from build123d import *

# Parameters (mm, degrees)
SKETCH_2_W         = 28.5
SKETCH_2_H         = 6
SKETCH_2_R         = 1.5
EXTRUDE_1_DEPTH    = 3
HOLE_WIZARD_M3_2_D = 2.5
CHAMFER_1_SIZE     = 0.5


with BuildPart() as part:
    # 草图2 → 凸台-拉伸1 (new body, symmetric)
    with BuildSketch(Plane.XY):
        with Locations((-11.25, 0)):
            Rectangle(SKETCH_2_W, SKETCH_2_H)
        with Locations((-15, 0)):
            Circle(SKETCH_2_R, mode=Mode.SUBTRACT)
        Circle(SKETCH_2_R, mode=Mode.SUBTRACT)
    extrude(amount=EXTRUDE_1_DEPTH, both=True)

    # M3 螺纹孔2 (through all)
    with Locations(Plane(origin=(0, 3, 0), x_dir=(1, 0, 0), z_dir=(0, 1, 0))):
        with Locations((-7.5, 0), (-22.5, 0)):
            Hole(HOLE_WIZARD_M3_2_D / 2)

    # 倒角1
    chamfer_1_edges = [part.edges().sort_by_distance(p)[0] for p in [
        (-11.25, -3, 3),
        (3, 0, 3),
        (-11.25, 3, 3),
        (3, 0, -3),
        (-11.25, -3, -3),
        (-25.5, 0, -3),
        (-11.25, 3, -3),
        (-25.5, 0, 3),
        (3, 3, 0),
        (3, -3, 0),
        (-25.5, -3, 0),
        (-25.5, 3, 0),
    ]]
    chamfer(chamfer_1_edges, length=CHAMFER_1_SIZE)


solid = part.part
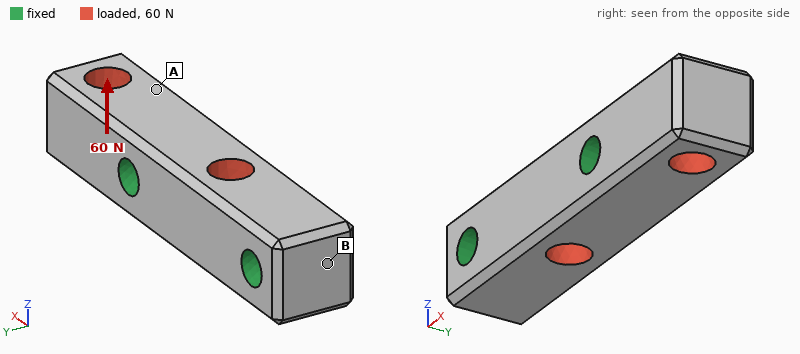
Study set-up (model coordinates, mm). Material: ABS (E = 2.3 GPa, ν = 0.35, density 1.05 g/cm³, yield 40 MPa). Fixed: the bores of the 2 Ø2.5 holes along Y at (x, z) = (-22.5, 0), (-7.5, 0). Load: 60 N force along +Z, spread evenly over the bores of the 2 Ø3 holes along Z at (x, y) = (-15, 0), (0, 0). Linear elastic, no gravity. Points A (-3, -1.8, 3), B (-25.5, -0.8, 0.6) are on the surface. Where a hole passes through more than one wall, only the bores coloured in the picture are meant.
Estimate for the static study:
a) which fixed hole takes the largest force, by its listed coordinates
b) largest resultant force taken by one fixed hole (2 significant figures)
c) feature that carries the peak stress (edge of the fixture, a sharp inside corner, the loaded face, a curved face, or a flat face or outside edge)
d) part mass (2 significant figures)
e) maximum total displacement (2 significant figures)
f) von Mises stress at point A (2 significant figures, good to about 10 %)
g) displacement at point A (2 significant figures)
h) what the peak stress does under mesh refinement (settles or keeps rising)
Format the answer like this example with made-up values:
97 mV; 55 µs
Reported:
(-7.5, 0); 49 N; edge of the fixture; 0.91 g; 47 µm; 2.9 MPa; 18 µm; keeps rising
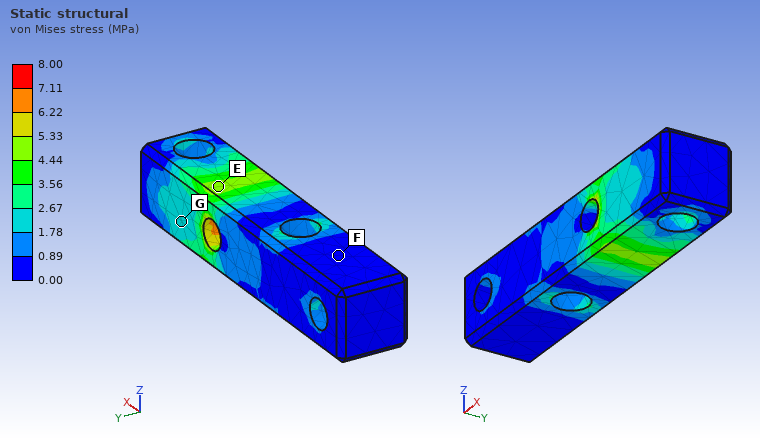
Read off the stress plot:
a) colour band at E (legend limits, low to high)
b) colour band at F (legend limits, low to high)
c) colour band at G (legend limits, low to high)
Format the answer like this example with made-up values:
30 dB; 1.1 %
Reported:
4.44 to 5.33 MPa; 0.00 to 0.89 MPa; 1.78 to 2.67 MPa
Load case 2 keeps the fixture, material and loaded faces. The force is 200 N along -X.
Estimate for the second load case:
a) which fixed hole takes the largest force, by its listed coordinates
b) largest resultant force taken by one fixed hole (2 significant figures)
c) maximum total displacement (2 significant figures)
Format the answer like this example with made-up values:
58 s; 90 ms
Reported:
(-7.5, 0); 150 N; 18 µm
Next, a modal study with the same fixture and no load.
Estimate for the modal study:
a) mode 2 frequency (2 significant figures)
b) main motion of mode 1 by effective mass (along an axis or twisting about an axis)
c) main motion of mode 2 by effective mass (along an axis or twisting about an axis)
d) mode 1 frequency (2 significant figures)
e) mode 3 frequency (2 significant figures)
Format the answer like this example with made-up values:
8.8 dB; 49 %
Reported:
12 kHz; along Z; along Y; 10 kHz; 21 kHz
